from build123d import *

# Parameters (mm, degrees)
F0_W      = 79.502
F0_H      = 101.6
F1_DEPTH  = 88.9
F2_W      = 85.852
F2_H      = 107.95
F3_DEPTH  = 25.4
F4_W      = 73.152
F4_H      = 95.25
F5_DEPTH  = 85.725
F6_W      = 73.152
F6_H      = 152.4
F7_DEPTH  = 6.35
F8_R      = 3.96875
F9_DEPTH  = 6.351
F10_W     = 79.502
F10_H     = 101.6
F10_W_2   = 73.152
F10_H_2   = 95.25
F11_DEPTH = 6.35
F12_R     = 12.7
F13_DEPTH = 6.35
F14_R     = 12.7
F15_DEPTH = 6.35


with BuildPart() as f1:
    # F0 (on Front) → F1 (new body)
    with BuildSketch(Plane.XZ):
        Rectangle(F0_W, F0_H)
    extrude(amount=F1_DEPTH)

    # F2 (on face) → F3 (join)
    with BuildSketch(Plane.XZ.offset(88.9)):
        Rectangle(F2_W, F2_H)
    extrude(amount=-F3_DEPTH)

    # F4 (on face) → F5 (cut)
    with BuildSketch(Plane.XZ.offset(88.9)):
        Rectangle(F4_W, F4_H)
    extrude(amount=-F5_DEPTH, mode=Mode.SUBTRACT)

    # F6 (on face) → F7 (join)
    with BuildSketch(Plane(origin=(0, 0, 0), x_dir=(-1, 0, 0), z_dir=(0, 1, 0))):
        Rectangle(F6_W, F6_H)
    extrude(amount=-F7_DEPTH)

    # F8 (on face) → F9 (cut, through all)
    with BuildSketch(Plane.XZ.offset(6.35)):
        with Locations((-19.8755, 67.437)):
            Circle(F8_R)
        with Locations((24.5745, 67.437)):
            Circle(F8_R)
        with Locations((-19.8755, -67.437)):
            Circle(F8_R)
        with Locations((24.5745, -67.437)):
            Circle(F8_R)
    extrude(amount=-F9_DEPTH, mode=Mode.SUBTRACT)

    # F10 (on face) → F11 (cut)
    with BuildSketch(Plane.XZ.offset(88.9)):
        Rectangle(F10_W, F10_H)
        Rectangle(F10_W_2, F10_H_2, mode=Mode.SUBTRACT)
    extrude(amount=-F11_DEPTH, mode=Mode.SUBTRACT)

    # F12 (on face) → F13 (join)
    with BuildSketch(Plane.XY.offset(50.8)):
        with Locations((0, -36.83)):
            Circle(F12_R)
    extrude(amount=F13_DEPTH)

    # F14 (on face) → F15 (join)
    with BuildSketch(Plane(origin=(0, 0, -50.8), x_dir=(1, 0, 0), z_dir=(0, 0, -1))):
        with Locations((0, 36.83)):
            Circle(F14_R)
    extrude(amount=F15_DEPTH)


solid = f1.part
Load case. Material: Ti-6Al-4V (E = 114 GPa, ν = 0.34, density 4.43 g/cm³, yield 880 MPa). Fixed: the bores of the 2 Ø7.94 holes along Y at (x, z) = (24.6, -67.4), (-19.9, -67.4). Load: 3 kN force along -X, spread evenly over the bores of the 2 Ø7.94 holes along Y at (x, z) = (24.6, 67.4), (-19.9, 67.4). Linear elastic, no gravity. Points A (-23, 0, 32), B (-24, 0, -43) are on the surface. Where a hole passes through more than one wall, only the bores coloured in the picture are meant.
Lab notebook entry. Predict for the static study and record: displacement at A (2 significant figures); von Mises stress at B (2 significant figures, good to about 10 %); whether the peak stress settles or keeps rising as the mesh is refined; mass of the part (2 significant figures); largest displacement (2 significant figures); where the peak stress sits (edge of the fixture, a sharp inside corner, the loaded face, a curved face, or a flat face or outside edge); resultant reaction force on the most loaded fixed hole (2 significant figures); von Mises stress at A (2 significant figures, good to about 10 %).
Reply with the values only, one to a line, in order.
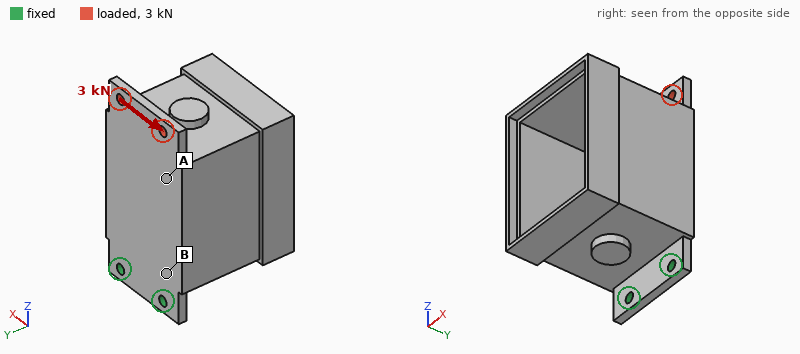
0.085 mm
36 MPa
keeps rising
860 g
0.14 mm
edge of the fixture
8.4 kN
12 MPa
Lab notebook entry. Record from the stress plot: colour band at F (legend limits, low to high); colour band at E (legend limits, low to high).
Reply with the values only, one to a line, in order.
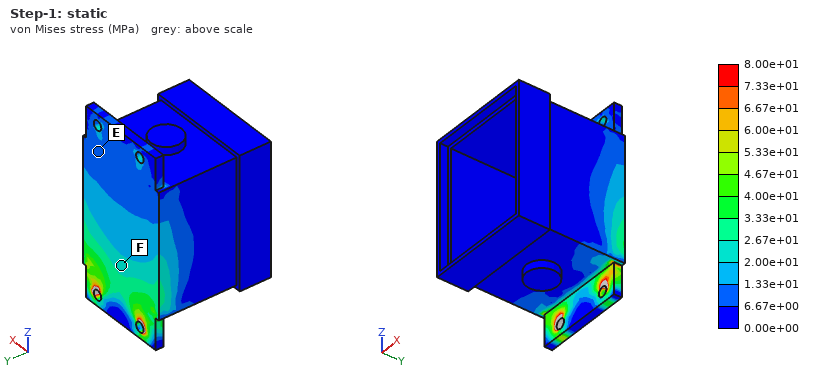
2.00e+01 to 2.67e+01 MPa
6.67e+00 to 1.33e+01 MPa
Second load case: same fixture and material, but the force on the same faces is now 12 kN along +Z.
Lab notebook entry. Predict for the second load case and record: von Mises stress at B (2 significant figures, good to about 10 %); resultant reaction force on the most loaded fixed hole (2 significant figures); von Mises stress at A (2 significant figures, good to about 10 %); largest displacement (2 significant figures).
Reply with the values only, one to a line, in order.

26 MPa
6.1 kN
23 MPa
54 µm
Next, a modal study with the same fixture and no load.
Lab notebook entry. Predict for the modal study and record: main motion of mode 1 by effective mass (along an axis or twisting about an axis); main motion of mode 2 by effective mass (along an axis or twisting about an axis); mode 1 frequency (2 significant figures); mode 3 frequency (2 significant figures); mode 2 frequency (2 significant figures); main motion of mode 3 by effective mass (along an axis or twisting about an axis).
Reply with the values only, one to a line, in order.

along Y
along X
180 Hz
1600 Hz
580 Hz
along X
